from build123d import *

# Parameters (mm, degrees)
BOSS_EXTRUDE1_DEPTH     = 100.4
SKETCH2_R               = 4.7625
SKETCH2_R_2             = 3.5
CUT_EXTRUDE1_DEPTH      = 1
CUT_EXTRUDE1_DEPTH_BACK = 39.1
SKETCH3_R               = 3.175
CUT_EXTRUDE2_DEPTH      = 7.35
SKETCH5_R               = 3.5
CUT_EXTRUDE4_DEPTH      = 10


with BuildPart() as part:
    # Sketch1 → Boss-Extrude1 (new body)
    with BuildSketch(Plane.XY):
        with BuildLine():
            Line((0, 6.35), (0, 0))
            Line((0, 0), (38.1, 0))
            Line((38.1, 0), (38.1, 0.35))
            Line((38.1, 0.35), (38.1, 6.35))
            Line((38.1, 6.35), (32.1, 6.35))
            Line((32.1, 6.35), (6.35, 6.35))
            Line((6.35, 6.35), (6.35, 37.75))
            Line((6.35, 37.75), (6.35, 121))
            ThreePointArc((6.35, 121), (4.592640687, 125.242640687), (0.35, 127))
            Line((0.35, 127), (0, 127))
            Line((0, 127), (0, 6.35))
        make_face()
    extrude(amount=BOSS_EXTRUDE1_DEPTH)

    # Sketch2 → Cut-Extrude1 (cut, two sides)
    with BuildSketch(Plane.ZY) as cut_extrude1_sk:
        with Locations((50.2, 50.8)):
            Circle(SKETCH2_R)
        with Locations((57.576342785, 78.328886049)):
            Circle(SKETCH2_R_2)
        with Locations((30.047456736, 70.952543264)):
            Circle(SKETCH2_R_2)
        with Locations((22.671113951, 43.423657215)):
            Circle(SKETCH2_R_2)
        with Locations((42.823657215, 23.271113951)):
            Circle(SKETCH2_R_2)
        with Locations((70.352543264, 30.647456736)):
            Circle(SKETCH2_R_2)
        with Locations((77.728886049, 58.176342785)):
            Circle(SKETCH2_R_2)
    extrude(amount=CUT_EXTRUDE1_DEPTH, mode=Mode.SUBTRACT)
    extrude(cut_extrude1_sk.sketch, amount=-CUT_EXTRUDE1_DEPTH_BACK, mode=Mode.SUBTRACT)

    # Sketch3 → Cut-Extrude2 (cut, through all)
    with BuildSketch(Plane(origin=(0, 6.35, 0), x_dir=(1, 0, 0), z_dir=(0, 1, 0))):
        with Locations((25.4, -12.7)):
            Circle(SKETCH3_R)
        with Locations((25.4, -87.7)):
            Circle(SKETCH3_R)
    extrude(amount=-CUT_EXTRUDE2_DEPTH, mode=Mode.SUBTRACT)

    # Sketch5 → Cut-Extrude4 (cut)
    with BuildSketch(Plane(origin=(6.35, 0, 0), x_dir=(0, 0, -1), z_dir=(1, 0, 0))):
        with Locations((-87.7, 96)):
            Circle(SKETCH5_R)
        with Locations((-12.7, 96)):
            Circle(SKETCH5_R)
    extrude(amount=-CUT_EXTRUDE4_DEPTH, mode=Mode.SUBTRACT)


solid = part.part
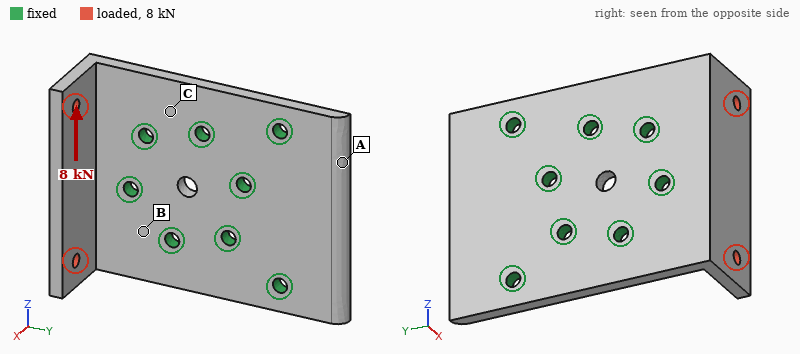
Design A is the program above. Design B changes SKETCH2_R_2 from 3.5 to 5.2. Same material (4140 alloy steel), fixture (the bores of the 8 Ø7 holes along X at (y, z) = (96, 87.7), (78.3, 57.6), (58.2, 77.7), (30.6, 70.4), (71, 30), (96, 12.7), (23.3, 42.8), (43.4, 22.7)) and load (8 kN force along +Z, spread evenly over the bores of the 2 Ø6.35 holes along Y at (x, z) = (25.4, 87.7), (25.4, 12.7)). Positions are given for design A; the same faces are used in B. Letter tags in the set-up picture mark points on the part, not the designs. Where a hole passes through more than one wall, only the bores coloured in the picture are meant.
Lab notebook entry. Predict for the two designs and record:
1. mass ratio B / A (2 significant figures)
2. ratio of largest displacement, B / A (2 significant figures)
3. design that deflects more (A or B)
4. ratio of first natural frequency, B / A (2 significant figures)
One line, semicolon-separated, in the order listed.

0.98; 0.86; A; 1.1
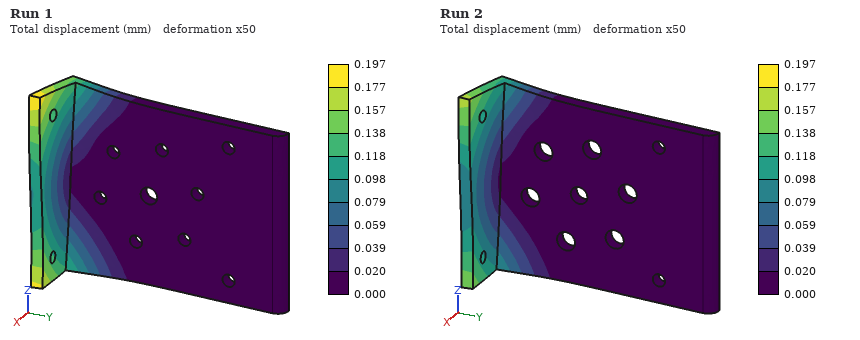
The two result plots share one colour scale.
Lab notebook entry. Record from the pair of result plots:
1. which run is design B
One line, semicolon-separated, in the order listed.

Run 2
